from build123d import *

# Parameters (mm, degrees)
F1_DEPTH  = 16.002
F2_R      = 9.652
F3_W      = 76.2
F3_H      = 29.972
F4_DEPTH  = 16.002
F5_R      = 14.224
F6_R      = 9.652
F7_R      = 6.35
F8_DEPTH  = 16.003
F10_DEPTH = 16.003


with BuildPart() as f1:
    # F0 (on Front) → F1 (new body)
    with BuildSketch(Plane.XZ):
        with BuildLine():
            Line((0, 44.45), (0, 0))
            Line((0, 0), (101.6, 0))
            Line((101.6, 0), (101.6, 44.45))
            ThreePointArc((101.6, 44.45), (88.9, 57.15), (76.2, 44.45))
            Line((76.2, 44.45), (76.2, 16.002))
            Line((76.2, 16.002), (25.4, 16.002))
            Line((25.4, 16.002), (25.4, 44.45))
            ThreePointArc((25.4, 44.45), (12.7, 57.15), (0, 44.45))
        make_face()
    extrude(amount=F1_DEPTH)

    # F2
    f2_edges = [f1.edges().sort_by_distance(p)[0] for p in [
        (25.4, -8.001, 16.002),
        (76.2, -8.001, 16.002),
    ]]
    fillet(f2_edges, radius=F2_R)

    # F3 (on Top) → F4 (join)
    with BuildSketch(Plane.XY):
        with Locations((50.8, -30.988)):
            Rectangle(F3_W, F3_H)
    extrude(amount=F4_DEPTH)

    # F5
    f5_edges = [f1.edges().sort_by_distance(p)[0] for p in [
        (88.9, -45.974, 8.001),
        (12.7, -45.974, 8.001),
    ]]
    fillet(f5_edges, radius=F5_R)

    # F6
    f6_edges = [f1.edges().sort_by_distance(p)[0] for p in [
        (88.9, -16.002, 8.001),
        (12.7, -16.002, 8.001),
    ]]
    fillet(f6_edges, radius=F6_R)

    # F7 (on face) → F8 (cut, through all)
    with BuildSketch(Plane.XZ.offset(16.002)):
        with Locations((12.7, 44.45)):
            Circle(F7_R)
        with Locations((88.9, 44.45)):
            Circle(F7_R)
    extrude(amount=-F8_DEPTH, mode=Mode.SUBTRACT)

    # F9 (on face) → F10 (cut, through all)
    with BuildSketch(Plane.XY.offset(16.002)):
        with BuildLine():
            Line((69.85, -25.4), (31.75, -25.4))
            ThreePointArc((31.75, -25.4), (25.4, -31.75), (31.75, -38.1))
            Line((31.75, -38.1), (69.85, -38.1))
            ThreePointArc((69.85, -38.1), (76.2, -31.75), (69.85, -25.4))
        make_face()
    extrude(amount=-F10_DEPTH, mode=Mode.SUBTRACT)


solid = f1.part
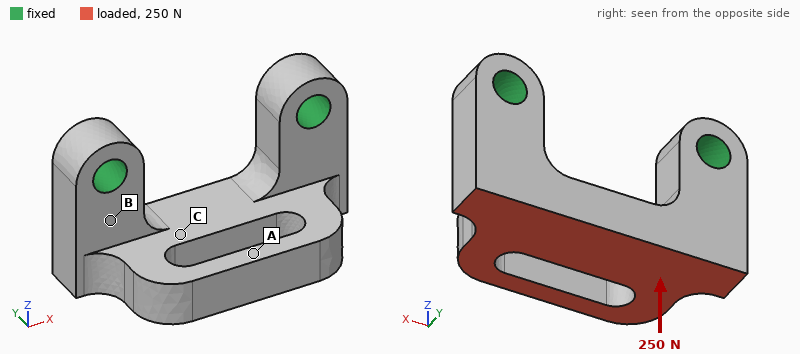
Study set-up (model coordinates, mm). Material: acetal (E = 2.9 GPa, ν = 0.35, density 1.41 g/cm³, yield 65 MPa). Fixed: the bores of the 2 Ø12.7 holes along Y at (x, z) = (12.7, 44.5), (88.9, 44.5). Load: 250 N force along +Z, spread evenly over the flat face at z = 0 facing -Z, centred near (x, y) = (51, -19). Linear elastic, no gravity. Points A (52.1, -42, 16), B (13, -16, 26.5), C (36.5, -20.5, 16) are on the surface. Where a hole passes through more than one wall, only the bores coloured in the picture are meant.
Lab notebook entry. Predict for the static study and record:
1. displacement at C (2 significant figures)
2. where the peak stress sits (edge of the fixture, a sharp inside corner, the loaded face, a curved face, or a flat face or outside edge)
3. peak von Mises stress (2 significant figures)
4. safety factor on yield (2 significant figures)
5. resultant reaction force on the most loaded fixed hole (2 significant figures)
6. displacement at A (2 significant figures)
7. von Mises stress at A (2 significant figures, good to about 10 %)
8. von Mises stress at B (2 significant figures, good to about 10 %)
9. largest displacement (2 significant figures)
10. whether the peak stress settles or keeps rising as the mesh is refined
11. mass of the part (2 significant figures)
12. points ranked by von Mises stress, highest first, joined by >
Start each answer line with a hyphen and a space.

- 0.034 mm
- a curved face
- 2.7 MPa
- 24
- 130 N
- 0.087 mm
- 0.64 MPa
- 1.6 MPa
- 0.11 mm
- settles
- 110 g
- B > A > C
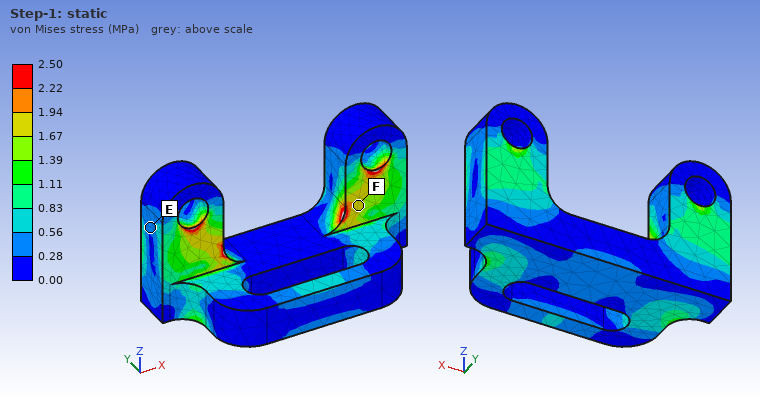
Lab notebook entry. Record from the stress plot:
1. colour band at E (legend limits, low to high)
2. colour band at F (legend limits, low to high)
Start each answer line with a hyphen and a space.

- 0.28 to 0.56 MPa
- 1.67 to 1.94 MPa
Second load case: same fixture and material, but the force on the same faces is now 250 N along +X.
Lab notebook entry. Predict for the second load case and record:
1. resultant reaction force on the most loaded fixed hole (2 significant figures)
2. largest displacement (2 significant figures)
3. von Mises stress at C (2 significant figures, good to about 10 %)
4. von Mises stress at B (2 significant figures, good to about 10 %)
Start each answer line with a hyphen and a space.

- 150 N
- 39 µm
- 0.54 MPa
- 0.95 MPa
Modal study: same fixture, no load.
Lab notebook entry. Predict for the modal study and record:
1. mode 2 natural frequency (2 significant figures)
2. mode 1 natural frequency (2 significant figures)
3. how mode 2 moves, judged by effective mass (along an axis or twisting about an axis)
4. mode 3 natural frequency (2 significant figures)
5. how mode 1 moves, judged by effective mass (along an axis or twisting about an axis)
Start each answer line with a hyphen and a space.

- 1500 Hz
- 850 Hz
- along X
- 2000 Hz
- along Y
